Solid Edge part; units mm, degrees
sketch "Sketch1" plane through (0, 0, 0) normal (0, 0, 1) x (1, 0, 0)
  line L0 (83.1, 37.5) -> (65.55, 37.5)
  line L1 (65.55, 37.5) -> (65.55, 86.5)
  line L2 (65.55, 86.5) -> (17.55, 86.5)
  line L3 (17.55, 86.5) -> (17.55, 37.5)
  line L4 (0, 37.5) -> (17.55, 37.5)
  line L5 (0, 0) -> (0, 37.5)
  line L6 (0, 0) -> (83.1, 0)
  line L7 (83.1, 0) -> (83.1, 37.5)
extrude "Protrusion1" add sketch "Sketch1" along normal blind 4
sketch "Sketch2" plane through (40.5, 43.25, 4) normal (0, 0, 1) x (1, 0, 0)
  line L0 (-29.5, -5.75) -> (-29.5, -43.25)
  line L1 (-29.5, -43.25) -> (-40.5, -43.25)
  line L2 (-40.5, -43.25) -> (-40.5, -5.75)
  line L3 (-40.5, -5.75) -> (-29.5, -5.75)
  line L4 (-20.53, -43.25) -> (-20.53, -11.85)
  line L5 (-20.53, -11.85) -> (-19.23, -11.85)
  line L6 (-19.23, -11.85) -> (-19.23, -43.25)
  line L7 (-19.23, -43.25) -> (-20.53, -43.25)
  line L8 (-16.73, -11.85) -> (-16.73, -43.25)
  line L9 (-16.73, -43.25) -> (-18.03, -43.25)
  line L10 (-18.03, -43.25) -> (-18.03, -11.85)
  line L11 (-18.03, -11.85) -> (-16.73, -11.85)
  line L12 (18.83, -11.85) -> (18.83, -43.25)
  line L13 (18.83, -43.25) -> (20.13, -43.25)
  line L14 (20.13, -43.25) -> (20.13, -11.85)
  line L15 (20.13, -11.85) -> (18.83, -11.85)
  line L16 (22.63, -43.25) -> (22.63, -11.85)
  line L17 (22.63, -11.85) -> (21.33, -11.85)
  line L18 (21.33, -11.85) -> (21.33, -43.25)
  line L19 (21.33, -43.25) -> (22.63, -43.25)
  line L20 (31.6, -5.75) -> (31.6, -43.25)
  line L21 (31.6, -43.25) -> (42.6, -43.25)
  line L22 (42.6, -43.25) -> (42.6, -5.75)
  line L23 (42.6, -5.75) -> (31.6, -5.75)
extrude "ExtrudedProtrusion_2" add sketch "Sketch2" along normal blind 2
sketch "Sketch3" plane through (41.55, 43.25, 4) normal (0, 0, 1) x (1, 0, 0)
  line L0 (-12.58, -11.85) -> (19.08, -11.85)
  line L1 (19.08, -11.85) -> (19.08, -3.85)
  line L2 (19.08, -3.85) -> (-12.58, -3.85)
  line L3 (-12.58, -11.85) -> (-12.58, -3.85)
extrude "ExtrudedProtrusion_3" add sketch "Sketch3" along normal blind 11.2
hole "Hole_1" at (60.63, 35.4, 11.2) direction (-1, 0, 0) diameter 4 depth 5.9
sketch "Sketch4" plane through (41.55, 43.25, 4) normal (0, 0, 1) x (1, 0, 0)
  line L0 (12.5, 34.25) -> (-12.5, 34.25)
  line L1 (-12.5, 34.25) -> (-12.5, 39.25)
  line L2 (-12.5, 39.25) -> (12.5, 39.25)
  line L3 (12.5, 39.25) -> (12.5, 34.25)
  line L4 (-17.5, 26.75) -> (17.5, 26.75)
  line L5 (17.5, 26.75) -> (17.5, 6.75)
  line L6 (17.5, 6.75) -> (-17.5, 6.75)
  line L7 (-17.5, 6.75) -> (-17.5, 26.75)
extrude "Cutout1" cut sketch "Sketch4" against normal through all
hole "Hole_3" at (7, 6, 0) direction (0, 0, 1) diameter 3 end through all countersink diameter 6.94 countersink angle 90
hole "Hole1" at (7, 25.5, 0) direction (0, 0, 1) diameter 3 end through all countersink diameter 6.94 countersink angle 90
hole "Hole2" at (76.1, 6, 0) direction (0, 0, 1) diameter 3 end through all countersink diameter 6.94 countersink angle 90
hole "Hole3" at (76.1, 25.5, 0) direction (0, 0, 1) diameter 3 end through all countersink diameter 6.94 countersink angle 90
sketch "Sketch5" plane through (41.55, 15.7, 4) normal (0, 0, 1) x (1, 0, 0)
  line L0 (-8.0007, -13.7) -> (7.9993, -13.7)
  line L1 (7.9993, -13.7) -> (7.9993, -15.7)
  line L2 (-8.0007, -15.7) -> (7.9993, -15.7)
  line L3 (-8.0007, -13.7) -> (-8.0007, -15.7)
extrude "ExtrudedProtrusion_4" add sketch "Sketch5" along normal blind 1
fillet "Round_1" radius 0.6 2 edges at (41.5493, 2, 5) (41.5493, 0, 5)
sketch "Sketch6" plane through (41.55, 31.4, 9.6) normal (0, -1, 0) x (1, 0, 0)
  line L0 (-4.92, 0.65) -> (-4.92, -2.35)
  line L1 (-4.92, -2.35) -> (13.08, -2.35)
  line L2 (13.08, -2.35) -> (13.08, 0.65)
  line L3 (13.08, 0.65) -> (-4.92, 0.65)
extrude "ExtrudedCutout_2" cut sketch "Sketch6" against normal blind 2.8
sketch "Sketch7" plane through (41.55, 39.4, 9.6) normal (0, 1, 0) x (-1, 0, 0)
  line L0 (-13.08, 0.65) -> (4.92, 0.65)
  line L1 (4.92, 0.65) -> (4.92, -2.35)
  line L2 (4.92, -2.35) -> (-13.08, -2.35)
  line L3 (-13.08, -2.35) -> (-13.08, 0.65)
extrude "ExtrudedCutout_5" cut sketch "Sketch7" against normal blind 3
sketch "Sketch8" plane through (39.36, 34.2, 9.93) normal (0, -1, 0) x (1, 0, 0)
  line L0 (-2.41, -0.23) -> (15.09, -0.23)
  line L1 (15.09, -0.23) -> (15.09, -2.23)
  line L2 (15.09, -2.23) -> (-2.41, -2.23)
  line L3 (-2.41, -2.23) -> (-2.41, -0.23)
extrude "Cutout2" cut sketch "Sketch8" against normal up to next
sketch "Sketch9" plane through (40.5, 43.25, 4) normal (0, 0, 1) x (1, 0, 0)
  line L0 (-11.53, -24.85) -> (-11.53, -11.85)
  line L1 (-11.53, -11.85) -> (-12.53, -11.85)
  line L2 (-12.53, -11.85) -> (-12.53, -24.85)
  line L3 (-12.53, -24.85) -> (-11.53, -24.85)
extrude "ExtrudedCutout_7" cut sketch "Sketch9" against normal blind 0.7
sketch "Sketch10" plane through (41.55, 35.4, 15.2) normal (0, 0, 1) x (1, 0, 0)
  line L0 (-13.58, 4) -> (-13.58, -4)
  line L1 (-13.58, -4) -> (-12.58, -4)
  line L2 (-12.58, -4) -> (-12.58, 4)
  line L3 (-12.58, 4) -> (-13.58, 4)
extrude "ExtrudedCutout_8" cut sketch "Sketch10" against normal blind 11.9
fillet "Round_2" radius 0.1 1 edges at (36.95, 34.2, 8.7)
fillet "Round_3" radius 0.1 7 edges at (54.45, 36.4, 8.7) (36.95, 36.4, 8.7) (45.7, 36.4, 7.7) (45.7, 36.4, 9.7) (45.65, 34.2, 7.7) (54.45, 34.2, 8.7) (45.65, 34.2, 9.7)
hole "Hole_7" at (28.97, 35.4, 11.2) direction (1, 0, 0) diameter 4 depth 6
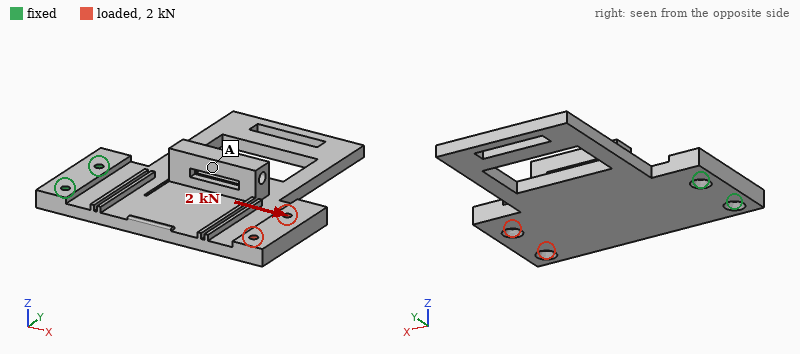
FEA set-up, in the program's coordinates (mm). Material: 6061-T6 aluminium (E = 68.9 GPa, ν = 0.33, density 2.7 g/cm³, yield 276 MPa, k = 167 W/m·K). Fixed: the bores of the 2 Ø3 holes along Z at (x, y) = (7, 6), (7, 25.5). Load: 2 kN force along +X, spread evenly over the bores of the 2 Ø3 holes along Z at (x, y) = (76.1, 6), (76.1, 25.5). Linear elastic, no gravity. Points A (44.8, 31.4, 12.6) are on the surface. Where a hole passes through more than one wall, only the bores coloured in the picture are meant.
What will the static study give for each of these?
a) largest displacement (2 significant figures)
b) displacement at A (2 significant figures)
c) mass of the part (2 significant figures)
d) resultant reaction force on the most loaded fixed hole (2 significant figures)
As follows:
0.54 mm
0.19 mm
61 g
1.0 kN
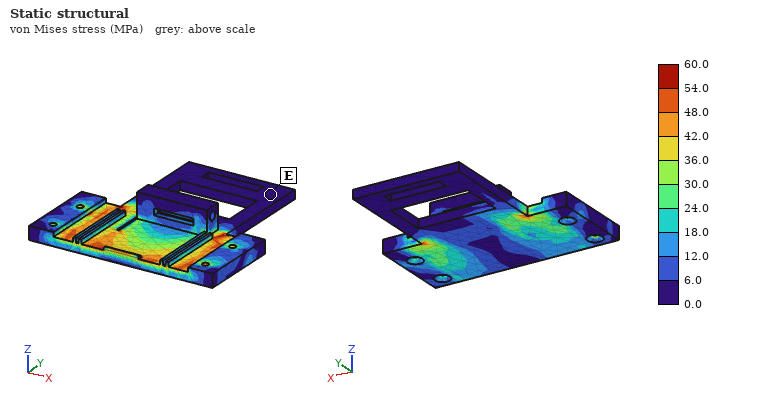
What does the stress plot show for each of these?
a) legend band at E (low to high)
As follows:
0.0 to 6.0 MPa
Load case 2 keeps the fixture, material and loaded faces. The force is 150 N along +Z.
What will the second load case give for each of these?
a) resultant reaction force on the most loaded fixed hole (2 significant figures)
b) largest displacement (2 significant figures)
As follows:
130 N
1.1 mm
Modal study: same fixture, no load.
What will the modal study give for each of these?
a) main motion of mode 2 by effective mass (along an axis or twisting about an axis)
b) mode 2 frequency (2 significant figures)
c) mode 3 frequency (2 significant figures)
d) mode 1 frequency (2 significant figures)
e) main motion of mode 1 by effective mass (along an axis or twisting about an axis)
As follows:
twisting about X
750 Hz
2000 Hz
450 Hz
along Z
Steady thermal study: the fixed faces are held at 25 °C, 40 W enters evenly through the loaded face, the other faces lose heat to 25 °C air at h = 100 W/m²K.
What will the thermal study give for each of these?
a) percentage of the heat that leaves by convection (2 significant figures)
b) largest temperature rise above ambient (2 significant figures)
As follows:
65 %
60 K
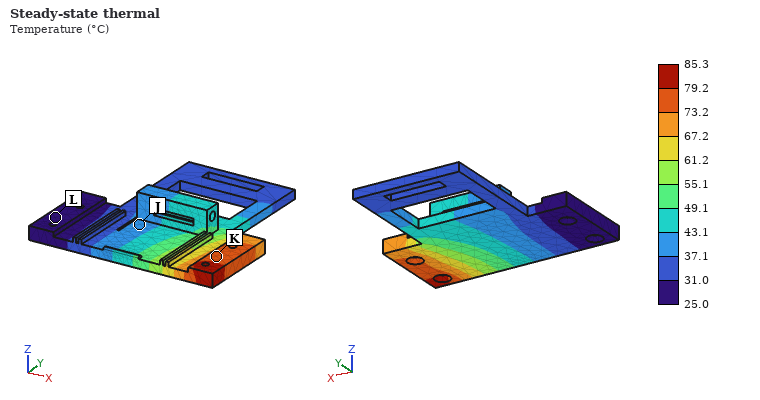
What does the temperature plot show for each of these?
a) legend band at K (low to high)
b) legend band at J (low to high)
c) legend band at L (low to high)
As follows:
73.2 to 79.2 °C
37.1 to 43.1 °C
25.0 to 31.0 °C
